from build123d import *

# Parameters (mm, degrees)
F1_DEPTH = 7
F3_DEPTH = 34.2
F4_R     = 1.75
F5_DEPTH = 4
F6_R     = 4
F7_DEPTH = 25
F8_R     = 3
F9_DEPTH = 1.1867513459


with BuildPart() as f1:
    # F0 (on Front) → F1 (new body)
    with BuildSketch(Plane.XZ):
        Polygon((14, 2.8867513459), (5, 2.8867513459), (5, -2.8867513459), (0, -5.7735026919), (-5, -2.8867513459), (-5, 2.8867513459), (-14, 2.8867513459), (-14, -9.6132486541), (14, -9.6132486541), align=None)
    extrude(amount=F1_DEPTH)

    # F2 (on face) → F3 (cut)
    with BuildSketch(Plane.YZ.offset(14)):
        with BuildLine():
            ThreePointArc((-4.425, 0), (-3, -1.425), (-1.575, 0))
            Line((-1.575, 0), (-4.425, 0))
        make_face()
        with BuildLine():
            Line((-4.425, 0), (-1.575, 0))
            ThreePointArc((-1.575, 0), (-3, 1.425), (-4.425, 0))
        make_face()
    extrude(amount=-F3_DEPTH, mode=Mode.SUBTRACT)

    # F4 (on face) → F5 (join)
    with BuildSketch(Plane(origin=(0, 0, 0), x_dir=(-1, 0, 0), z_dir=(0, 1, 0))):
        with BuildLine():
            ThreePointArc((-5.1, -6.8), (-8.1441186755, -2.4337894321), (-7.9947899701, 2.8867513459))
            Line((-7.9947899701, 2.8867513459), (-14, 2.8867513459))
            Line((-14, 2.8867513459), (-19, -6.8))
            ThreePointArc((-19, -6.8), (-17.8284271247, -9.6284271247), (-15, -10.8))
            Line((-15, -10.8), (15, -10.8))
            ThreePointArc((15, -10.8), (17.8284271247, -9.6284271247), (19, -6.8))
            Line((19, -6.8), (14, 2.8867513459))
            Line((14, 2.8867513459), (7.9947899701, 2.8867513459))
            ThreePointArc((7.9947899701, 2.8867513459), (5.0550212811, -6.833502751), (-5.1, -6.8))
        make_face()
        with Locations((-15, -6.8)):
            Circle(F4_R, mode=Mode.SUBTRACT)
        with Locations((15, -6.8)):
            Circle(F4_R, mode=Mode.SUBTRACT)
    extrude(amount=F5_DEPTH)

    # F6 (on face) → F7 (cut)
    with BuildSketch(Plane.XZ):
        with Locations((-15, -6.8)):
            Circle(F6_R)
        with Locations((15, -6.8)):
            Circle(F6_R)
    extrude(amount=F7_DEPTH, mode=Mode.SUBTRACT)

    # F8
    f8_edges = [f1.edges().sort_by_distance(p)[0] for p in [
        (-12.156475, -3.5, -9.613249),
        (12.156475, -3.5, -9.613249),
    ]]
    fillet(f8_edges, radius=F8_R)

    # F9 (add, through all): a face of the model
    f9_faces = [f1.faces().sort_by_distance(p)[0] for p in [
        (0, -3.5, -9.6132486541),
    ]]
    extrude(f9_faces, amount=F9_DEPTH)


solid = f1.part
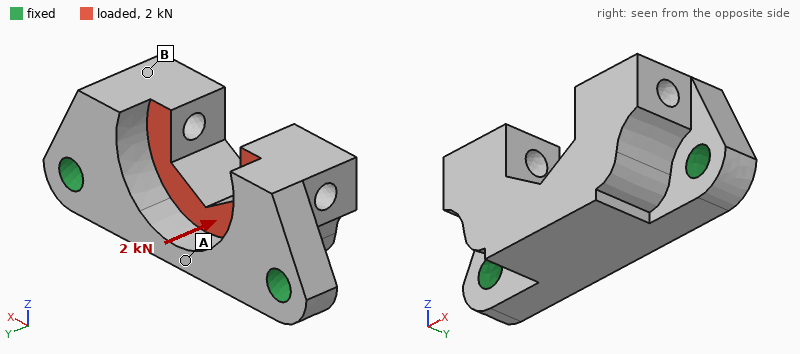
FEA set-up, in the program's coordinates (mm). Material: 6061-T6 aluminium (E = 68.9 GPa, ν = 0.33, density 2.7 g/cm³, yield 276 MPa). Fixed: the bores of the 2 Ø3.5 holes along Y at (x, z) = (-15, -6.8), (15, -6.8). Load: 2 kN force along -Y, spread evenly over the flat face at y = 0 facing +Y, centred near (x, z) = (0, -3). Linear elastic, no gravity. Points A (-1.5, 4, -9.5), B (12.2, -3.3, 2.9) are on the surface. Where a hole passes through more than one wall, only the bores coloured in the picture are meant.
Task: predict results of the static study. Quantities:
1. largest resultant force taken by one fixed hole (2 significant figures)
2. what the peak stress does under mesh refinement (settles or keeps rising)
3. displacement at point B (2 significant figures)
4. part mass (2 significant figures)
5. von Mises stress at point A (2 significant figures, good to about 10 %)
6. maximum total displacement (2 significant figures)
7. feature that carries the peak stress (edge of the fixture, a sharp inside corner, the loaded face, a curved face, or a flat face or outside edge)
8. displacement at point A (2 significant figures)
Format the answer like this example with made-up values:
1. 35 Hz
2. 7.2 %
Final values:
1. 1.2 kN
2. keeps rising
3. 32 µm
4. 7.6 g
5. 39 MPa
6. 48 µm
7. edge of the fixture
8. 9.8 µm
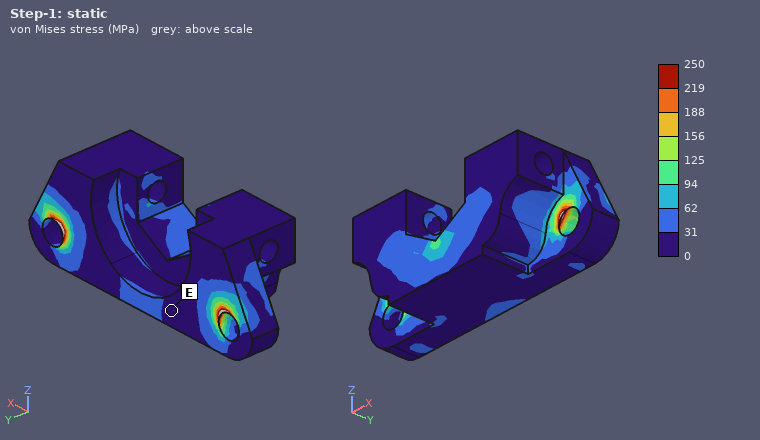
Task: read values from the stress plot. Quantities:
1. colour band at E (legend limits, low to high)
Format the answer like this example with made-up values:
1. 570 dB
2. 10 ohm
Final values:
1. 0 to 31 MPa
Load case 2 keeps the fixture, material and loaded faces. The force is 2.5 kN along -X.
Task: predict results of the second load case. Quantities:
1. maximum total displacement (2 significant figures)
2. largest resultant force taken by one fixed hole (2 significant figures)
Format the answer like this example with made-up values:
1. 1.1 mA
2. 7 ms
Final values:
1. 16 µm
2. 1.3 kN
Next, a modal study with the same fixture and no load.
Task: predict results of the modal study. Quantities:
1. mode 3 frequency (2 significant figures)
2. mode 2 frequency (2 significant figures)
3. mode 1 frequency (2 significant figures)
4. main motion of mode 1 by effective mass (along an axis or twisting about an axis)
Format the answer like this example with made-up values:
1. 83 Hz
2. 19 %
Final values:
1. 23 kHz
2. 22 kHz
3. 14 kHz
4. along Z
